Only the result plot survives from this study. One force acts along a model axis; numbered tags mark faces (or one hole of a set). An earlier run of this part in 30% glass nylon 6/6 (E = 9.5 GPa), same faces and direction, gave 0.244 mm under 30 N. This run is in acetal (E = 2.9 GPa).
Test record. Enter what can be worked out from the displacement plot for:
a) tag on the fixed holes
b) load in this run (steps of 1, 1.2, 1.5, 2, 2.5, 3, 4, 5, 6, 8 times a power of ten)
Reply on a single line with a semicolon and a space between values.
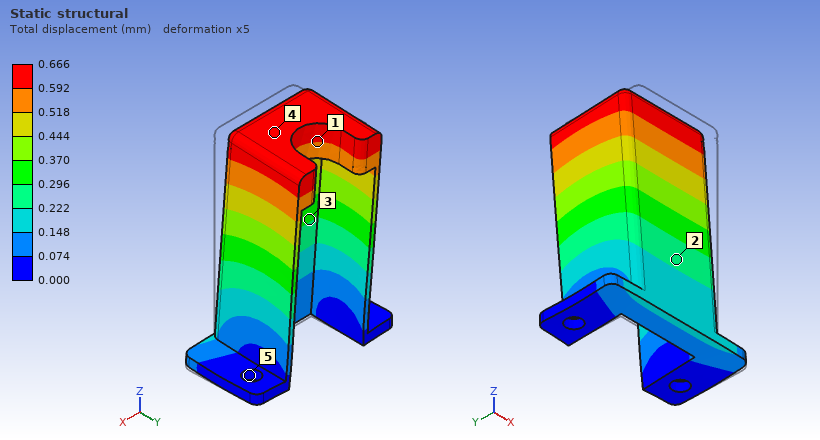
5; 25 N
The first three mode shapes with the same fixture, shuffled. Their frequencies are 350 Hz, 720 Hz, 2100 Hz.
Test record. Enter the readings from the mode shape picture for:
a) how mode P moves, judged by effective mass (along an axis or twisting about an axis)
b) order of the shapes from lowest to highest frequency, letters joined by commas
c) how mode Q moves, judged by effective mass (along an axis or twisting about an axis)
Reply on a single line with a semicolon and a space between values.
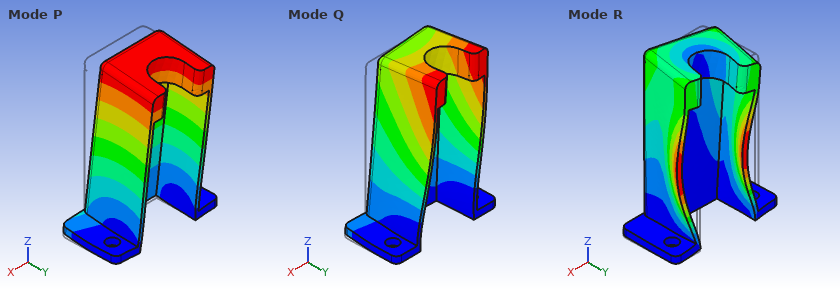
along Y; P, Q, R; along X
